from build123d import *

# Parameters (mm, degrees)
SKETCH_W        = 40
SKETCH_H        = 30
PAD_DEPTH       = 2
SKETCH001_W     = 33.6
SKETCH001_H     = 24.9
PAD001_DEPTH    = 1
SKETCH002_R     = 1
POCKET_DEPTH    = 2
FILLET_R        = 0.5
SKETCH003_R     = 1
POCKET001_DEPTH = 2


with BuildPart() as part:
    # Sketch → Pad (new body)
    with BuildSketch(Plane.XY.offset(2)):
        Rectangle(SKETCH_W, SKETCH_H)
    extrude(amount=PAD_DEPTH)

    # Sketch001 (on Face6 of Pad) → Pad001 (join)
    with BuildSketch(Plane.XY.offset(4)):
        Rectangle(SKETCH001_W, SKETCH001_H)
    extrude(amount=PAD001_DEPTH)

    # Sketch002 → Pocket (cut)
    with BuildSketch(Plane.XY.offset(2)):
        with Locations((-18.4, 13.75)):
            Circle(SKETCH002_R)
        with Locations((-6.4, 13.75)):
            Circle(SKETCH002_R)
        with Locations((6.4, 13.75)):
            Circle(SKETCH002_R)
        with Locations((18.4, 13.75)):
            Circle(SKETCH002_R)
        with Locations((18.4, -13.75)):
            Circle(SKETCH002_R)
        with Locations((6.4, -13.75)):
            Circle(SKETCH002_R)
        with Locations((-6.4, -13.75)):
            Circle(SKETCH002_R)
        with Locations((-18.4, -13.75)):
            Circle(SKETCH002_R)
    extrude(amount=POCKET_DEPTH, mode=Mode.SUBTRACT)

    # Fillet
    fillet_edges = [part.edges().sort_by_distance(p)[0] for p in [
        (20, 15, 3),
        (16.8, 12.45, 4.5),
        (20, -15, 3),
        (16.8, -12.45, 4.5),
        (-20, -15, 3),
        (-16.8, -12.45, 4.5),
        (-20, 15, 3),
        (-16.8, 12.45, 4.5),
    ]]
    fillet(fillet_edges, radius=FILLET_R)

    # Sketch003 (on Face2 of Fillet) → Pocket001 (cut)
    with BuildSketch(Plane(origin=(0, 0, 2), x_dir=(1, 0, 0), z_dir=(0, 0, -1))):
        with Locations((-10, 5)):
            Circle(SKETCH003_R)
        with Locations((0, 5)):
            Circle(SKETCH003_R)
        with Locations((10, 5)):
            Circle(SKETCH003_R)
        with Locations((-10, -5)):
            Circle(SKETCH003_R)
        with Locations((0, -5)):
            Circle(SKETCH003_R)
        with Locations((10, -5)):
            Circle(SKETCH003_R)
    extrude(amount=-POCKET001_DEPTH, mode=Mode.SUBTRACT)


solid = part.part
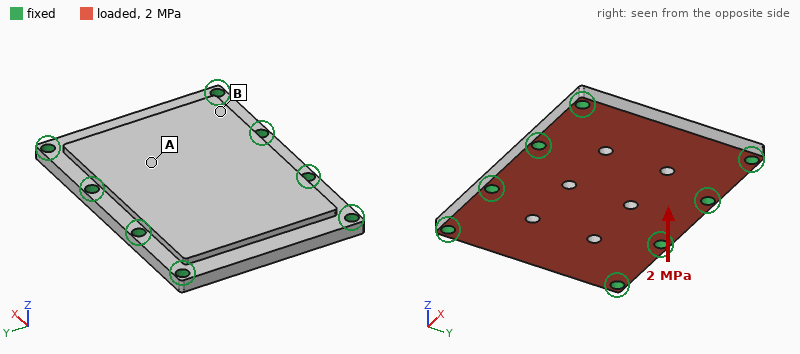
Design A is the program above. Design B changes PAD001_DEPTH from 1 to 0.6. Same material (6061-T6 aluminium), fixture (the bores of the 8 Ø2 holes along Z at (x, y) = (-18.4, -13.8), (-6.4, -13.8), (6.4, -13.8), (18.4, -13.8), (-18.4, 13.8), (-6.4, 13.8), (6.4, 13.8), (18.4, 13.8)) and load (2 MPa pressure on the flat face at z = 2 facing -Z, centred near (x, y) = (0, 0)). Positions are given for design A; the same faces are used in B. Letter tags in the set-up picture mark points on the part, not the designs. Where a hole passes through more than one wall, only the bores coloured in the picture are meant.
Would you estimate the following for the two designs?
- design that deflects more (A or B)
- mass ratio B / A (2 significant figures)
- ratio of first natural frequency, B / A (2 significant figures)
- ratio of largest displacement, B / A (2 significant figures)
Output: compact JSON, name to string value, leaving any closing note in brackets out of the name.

{"design that deflects more": "B", "mass ratio B / A": "0.89", "ratio of first natural frequency, B / A": "0.95", "ratio of largest displacement, B / A": "1.2"}
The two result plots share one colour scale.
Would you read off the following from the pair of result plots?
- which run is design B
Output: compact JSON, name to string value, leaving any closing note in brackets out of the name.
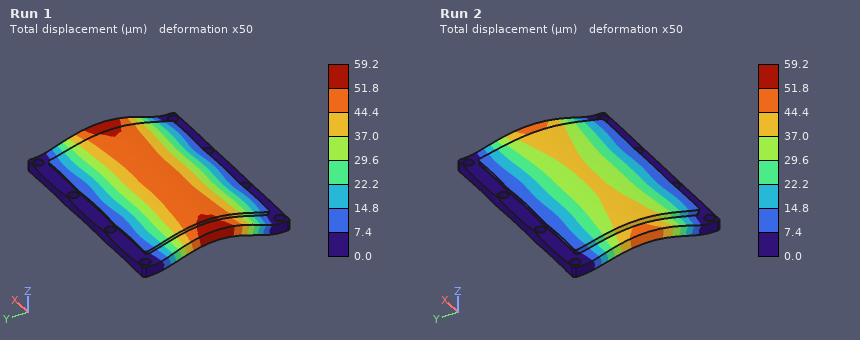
{"which run is design B": "Run 1"}
